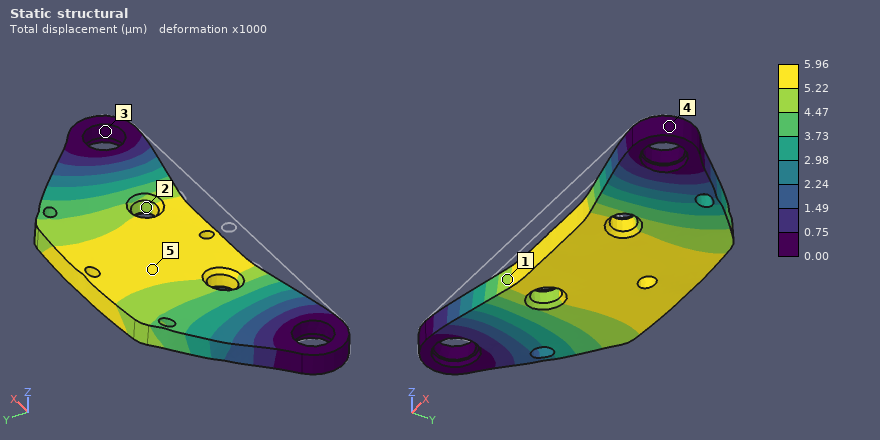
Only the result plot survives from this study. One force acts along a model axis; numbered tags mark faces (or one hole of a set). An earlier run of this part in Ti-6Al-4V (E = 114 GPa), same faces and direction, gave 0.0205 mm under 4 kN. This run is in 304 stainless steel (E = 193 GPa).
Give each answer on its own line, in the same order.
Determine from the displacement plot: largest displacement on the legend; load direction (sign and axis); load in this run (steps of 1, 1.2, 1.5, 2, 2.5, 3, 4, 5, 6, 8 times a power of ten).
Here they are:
5.96 µm
+Y
2 kN
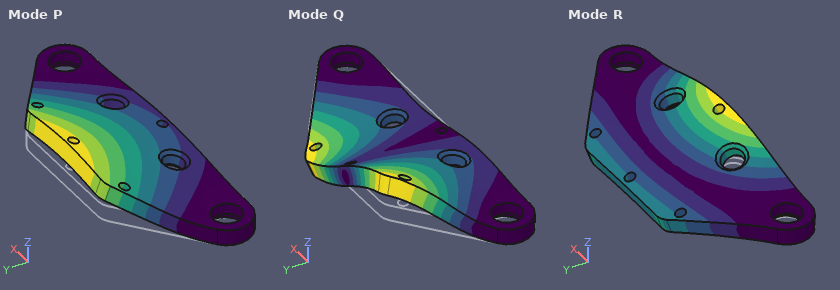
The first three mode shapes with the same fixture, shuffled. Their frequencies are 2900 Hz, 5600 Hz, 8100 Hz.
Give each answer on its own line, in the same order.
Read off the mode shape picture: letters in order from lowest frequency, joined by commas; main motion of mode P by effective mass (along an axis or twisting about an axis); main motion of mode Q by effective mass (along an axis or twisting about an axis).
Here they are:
P, R, Q
along Z
twisting about Y
